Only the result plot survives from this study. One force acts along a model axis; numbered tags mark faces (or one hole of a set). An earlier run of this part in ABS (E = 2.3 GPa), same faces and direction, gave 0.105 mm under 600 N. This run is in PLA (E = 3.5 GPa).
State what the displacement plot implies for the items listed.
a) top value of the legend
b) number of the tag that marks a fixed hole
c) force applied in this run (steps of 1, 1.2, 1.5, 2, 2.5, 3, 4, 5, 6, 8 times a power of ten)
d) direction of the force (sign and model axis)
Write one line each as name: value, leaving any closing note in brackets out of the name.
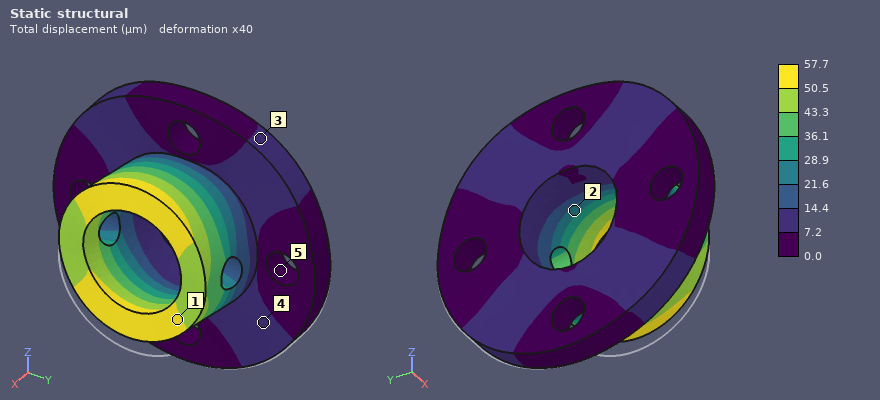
top value of the legend: 57.7 µm
number of the tag that marks a fixed hole: 5
force applied in this run: 500 N
direction of the force: +Z
